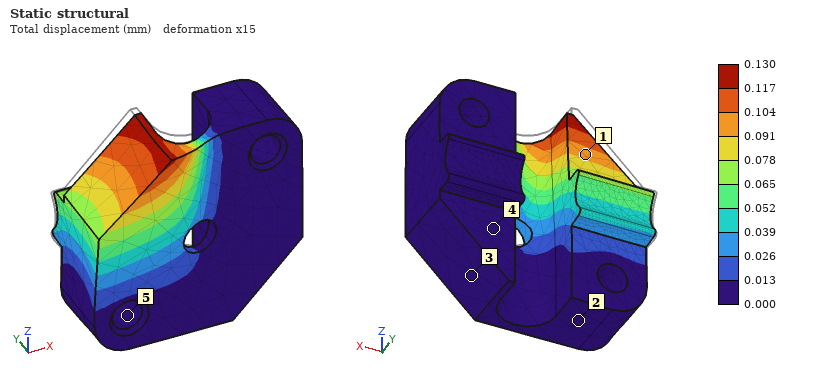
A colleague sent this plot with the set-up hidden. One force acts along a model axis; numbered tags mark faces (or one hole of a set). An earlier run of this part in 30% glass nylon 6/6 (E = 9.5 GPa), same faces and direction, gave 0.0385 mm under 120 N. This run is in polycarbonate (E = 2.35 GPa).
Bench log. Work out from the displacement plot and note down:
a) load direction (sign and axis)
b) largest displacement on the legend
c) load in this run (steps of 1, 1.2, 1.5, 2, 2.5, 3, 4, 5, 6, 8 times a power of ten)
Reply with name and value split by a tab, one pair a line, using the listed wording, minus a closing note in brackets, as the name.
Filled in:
load direction	-Y
largest displacement on the legend	0.130 mm
load in this run	100 N
